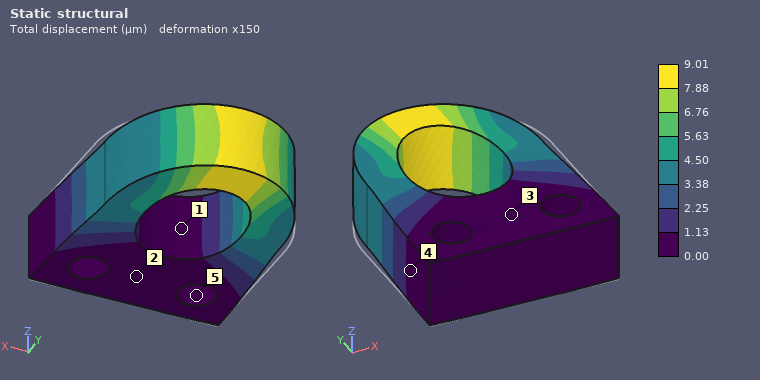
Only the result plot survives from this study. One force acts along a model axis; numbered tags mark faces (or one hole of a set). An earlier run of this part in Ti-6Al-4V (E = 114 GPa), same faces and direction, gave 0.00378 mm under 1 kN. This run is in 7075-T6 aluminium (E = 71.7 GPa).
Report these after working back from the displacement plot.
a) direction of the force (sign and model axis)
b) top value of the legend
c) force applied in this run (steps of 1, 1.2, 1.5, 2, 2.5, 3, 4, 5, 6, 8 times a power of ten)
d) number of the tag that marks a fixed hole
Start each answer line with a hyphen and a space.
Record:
- +Y
- 9.01 µm
- 1.5 kN
- 5
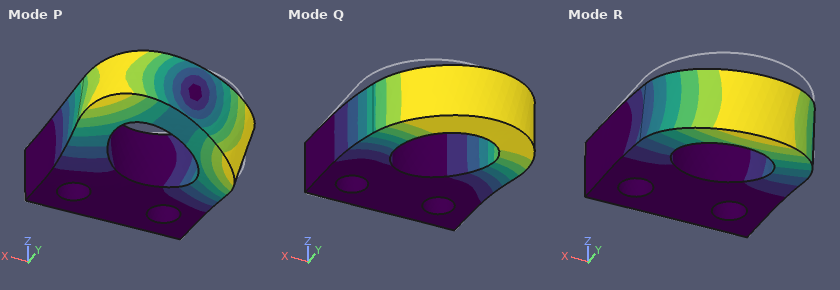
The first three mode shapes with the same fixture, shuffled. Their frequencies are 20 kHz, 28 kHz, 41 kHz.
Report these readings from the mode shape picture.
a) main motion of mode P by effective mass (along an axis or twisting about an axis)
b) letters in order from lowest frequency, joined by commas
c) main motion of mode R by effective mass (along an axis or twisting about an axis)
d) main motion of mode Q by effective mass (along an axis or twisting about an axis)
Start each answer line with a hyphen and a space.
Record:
- twisting about Y
- R, Q, P
- along Z
- along X
